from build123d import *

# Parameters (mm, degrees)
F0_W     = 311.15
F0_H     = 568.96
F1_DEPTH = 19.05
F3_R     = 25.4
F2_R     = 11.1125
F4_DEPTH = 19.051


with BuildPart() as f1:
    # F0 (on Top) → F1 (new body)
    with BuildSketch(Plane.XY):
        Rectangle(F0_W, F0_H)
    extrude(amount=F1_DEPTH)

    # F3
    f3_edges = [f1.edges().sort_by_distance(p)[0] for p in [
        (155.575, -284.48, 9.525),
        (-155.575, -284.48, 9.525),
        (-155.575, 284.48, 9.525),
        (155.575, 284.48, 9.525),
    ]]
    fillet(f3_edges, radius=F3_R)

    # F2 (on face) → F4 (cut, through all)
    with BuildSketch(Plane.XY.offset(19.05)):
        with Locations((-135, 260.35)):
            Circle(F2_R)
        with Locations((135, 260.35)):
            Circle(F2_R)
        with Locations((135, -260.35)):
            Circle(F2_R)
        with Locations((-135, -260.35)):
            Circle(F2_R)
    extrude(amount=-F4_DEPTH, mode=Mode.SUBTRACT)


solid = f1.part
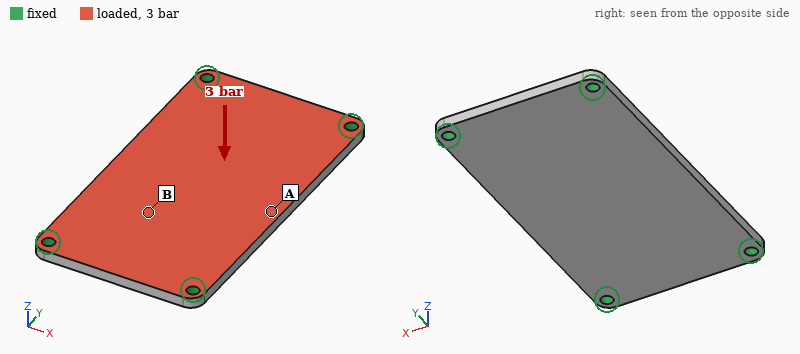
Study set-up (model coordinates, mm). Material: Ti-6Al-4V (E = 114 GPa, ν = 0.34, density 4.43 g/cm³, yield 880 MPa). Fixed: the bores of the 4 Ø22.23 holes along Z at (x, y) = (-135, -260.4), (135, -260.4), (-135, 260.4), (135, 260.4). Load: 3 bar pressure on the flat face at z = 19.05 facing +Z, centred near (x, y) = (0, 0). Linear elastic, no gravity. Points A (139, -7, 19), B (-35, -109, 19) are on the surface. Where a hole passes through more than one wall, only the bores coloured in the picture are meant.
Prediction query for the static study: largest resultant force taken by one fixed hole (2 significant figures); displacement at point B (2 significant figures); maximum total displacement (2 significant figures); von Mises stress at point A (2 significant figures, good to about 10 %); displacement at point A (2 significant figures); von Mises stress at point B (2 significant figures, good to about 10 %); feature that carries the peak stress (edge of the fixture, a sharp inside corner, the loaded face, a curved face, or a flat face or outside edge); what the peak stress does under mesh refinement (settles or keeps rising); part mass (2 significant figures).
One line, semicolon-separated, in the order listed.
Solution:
13 kN; 0.88 mm; 1.2 mm; 71 MPa; 1.2 mm; 34 MPa; edge of the fixture; keeps rising; 15 kg
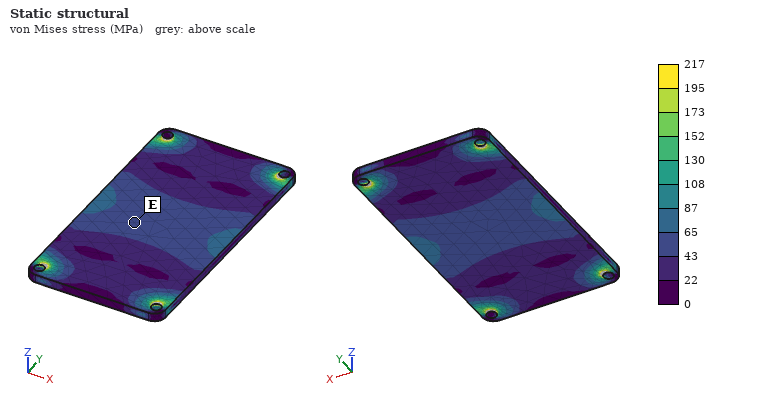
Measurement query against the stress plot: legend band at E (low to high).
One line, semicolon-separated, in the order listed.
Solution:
43 to 65 MPa
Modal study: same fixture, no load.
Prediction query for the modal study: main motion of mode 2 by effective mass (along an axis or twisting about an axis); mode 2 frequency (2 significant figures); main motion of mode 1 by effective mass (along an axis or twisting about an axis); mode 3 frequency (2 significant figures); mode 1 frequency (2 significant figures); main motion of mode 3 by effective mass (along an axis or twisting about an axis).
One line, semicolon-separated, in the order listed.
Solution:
twisting about Y; 540 Hz; along Z; 860 Hz; 310 Hz; twisting about X
